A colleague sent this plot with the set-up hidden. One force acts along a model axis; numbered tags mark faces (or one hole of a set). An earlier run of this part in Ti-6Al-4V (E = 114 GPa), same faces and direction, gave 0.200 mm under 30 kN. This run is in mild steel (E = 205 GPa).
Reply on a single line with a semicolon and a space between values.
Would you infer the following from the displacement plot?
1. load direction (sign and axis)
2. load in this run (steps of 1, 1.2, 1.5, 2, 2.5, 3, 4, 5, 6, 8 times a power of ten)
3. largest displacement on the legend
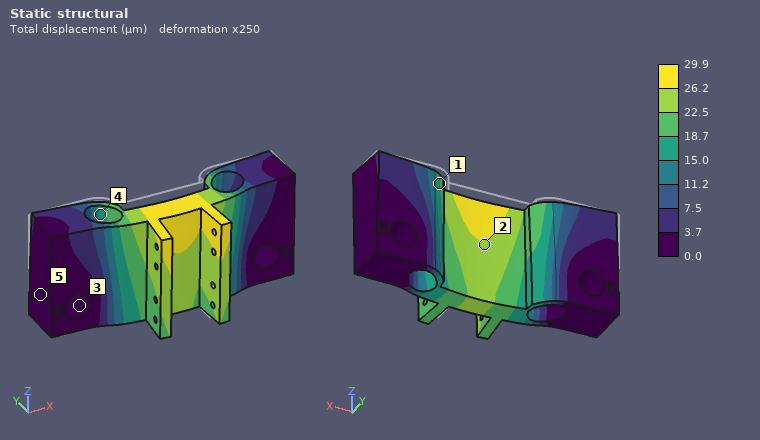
-Y; 8 kN; 29.9 µm
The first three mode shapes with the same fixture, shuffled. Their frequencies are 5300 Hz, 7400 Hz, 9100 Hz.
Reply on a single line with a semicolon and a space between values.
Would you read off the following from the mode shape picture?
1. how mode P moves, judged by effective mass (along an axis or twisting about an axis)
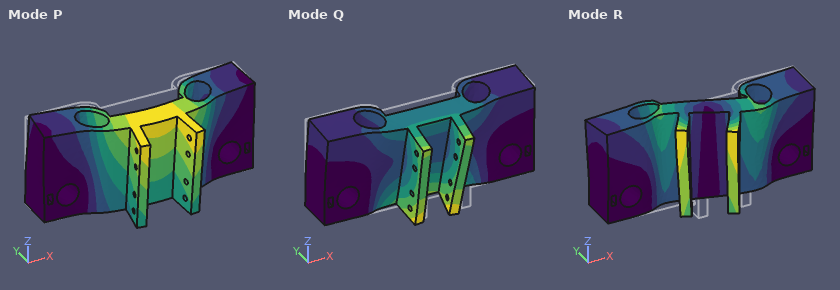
along Y
